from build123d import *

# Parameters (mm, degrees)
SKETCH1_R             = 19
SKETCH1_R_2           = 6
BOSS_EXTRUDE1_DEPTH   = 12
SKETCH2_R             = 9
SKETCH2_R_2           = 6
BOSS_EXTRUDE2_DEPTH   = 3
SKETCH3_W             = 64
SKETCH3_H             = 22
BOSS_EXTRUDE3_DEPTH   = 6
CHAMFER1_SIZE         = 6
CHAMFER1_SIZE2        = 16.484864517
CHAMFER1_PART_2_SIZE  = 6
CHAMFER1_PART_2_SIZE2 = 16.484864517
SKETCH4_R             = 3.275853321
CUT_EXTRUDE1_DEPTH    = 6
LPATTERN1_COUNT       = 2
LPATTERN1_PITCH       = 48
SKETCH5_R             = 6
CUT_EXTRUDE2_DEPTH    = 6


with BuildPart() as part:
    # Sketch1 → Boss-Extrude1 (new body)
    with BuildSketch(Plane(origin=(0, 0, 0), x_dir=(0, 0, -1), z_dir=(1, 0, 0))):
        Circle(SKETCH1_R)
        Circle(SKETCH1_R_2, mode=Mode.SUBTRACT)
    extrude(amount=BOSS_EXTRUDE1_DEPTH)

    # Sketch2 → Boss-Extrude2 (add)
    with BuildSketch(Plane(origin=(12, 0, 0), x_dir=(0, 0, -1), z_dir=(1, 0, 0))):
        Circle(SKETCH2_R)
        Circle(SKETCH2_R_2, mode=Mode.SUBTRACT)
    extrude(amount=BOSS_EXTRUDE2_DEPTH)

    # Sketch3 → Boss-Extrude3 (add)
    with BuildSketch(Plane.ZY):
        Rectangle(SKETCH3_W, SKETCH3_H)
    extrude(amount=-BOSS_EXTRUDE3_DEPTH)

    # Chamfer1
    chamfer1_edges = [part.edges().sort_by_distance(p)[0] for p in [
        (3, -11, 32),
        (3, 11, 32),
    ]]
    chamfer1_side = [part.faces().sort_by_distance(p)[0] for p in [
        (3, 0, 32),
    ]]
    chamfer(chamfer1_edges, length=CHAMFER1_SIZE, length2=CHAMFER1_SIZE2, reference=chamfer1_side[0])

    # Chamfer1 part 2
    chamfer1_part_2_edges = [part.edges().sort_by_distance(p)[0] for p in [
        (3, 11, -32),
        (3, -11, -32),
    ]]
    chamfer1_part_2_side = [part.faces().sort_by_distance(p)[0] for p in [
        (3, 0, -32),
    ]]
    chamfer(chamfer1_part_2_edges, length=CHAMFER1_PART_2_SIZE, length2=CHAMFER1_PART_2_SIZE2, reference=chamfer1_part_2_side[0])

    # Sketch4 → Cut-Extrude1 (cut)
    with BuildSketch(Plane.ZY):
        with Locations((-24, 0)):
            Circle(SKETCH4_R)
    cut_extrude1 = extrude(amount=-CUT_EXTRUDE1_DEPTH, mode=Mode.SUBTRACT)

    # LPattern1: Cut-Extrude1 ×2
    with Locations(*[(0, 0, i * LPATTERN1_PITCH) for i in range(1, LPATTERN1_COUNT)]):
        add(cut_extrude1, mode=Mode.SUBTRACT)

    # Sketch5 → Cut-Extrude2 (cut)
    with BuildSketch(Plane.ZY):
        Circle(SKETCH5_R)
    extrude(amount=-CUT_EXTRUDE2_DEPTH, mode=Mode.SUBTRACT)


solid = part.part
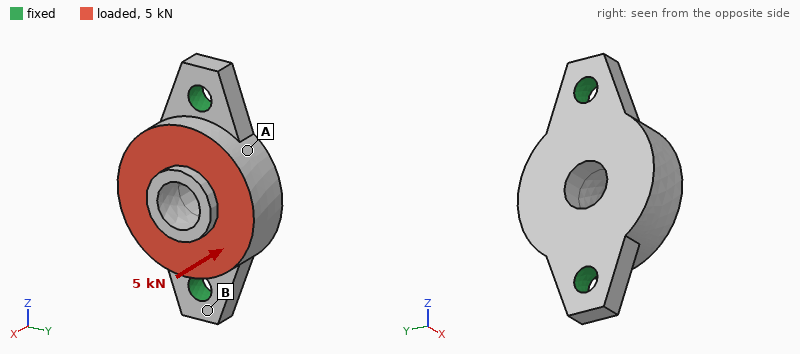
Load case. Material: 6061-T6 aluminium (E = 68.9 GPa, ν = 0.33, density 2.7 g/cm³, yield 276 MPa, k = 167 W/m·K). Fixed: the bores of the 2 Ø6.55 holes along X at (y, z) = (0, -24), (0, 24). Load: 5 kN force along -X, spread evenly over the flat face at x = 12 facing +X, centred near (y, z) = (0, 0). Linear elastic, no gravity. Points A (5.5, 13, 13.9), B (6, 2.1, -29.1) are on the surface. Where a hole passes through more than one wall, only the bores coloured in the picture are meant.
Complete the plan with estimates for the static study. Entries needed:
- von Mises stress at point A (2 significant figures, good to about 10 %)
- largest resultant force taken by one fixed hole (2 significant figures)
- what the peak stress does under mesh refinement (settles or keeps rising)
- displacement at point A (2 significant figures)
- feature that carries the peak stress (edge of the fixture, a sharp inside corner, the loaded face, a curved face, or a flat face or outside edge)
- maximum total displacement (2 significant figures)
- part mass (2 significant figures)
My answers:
29 MPa
2.9 kN
keeps rising
20 µm
edge of the fixture
32 µm
40 g
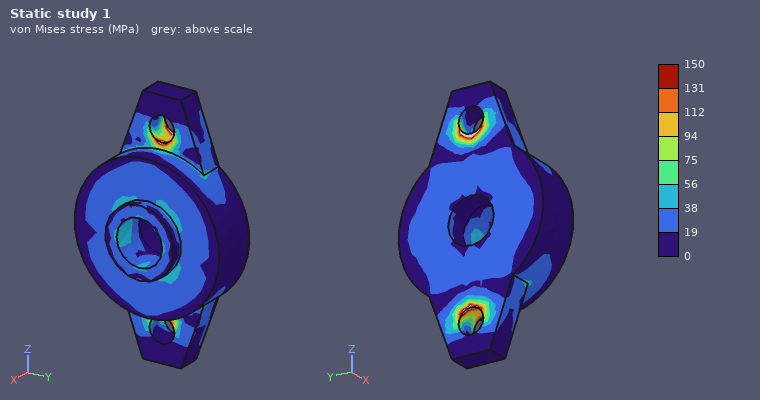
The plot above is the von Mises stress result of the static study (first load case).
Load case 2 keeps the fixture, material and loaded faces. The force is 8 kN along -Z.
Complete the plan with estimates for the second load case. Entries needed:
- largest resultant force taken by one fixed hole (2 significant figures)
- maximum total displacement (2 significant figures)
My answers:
4.4 kN
13 µm
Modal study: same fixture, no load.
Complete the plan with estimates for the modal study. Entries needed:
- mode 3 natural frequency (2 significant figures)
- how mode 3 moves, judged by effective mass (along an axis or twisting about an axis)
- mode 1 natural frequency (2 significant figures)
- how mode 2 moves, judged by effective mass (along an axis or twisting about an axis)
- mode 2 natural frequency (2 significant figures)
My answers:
21 kHz
along Y
8000 Hz
along X
13 kHz
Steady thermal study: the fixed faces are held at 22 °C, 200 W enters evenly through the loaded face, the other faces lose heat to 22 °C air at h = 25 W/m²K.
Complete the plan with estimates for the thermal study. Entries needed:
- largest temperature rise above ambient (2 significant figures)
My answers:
62 K
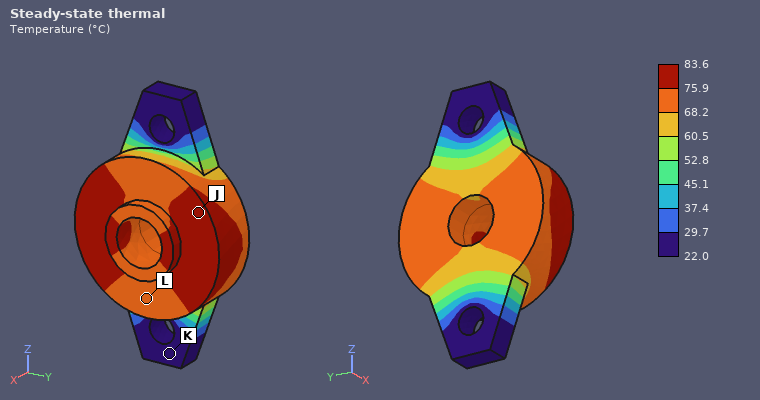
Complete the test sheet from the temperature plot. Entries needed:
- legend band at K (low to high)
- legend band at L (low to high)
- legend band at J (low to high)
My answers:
22.0 to 29.7 °C
68.2 to 75.9 °C
75.9 to 83.6 °C
